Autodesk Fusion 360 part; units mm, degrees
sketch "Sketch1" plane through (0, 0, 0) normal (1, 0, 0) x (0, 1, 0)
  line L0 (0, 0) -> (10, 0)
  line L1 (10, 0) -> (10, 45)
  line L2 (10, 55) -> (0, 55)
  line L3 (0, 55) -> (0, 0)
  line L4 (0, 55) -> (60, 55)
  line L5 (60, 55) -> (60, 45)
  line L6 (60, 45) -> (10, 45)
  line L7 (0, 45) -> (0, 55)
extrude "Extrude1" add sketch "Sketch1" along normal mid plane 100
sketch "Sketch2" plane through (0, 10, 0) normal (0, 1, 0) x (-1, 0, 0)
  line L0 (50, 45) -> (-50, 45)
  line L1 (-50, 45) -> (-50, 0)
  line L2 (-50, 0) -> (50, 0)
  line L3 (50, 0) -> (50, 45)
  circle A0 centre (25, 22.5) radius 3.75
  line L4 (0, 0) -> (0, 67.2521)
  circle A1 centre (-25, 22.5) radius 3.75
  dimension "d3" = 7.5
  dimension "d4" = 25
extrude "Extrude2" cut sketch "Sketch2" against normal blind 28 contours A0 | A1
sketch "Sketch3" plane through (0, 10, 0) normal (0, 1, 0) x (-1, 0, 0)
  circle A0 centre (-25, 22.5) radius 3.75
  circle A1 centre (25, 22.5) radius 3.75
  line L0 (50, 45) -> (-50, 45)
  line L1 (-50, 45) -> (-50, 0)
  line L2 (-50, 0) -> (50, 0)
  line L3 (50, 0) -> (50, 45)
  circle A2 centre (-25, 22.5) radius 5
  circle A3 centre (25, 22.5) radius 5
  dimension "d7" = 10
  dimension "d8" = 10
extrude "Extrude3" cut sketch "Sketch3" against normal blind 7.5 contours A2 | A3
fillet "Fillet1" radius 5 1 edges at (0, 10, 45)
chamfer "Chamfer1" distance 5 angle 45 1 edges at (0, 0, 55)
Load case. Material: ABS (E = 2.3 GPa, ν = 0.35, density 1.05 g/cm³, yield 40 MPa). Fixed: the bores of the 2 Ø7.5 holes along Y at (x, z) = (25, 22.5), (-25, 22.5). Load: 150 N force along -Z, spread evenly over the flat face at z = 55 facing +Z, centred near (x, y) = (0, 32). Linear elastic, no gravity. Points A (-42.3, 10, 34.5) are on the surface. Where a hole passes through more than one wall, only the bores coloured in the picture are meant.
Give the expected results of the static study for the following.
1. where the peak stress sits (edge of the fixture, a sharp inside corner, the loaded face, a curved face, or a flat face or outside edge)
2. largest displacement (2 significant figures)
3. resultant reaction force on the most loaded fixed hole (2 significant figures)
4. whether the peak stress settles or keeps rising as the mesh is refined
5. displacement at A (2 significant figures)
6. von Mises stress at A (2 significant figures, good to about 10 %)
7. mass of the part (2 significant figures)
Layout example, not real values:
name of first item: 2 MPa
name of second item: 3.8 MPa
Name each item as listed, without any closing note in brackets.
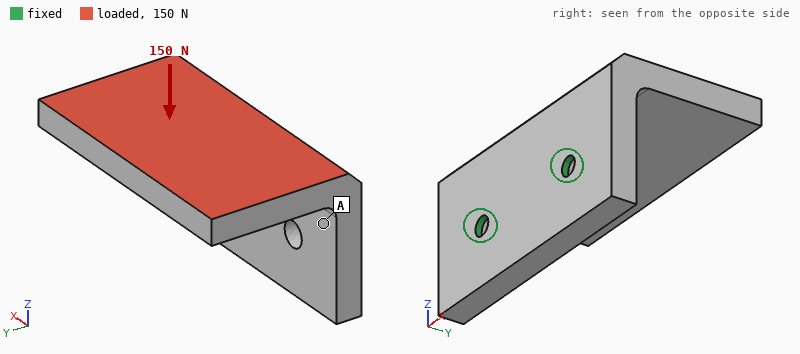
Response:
where the peak stress sits: edge of the fixture
largest displacement: 1.3 mm
resultant reaction force on the most loaded fixed hole: 75 N
whether the peak stress settles or keeps rising as the mesh is refined: keeps rising
displacement at A: 0.21 mm
von Mises stress at A: 2.5 MPa
mass of the part: 110 g
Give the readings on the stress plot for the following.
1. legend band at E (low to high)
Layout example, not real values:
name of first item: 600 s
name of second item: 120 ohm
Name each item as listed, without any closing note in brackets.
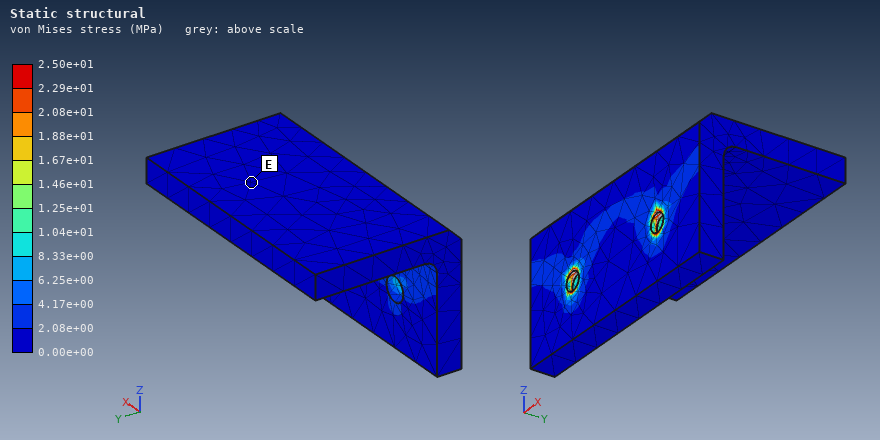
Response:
legend band at E: 0.00e+00 to 2.08e+00 MPa
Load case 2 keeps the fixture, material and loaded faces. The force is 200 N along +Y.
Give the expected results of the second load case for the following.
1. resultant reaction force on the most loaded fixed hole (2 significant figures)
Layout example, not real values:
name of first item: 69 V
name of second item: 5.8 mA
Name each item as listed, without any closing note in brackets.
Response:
resultant reaction force on the most loaded fixed hole: 100 N
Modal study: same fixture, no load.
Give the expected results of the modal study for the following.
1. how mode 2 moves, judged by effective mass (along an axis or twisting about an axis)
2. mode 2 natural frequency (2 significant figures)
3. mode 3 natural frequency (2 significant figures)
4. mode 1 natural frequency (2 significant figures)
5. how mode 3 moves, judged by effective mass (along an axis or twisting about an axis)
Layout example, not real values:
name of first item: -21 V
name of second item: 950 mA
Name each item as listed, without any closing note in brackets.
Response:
how mode 2 moves, judged by effective mass: along X
mode 2 natural frequency: 620 Hz
mode 3 natural frequency: 1100 Hz
mode 1 natural frequency: 240 Hz
how mode 3 moves, judged by effective mass: along Y
